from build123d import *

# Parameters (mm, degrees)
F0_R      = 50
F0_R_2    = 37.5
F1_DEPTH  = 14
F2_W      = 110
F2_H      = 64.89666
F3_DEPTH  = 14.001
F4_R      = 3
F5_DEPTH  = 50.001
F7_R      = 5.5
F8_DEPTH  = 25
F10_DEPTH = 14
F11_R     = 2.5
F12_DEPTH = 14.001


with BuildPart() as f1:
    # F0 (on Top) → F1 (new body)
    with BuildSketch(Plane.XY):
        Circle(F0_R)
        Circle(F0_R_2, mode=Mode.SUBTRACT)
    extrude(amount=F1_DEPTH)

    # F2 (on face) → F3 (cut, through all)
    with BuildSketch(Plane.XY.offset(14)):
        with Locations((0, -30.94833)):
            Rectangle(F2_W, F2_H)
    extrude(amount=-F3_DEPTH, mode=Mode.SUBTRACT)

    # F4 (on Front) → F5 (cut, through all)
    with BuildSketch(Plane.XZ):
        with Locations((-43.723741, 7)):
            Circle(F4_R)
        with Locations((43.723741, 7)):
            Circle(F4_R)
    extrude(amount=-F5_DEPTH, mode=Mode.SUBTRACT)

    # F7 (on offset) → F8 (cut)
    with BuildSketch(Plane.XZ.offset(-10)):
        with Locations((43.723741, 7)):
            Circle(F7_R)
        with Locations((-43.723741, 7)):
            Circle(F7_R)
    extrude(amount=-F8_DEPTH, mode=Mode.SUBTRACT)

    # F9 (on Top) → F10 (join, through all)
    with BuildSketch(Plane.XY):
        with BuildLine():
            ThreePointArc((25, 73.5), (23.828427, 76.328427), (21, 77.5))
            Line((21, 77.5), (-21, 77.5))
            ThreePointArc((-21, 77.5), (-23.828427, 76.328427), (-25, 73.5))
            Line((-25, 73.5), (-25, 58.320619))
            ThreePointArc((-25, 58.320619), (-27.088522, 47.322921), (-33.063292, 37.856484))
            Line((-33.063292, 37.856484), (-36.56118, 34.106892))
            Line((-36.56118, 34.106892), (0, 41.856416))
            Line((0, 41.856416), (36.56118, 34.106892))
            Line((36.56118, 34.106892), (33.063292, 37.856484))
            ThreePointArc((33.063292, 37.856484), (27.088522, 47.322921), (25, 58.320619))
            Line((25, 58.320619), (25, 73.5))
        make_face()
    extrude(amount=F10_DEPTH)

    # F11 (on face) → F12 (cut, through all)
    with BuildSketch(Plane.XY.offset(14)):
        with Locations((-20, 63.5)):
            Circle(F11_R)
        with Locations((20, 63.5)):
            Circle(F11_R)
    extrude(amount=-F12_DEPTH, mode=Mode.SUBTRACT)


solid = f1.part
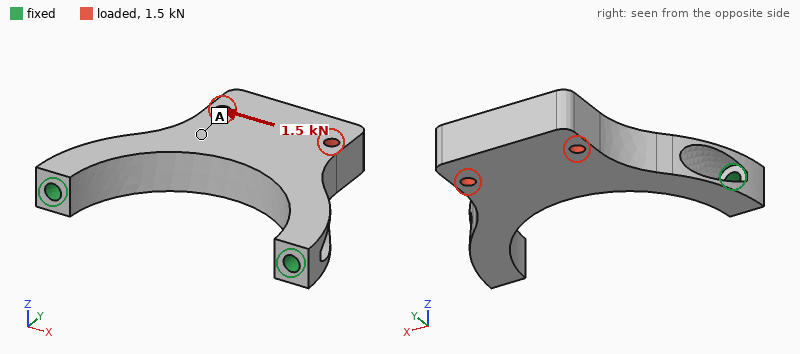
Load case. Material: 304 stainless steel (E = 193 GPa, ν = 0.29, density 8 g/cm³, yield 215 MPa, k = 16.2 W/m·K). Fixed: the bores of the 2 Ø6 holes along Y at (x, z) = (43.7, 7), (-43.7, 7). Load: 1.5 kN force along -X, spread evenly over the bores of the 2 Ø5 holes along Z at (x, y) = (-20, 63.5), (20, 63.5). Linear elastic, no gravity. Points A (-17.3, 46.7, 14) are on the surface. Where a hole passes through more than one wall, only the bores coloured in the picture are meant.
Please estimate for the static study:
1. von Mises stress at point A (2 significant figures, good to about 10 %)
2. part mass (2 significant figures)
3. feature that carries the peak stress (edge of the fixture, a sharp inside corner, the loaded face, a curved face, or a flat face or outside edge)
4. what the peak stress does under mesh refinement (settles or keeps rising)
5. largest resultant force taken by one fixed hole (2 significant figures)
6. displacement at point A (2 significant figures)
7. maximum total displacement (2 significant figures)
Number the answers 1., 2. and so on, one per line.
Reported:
1. 3.8 MPa
2. 330 g
3. edge of the fixture
4. keeps rising
5. 1.2 kN
6. 6.1 µm
7. 6.7 µm
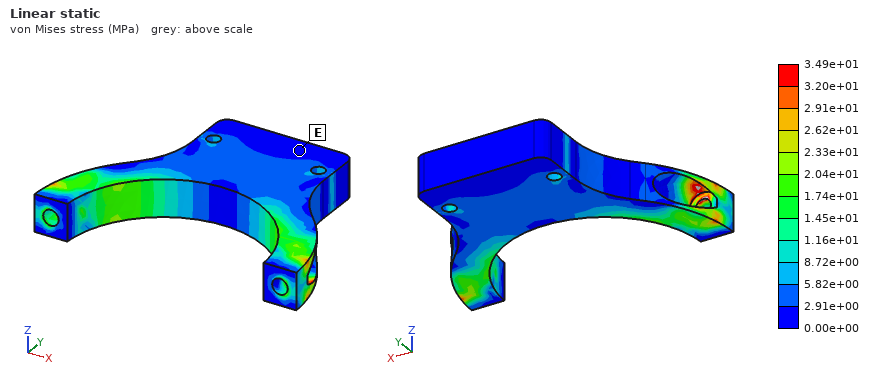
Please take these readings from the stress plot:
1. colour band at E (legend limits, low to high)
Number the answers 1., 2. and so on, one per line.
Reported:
1. 0.00e+00 to 2.91e+00 MPa
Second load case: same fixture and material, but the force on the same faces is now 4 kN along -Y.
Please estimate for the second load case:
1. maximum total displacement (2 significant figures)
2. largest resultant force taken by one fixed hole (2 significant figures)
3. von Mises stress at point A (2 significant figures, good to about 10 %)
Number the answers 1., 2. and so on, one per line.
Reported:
1. 7.1 µm
2. 2.2 kN
3. 6.9 MPa
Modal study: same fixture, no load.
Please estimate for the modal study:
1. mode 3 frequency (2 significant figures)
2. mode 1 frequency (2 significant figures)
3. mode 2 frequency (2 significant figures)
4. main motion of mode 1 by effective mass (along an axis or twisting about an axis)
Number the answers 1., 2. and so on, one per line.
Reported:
1. 4600 Hz
2. 1100 Hz
3. 4400 Hz
4. along Z
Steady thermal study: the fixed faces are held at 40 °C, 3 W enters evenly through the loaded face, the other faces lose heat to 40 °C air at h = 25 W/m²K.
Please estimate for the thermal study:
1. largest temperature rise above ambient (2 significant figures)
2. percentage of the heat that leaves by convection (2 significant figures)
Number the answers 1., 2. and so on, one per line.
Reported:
1. 14 K
2. 75 %
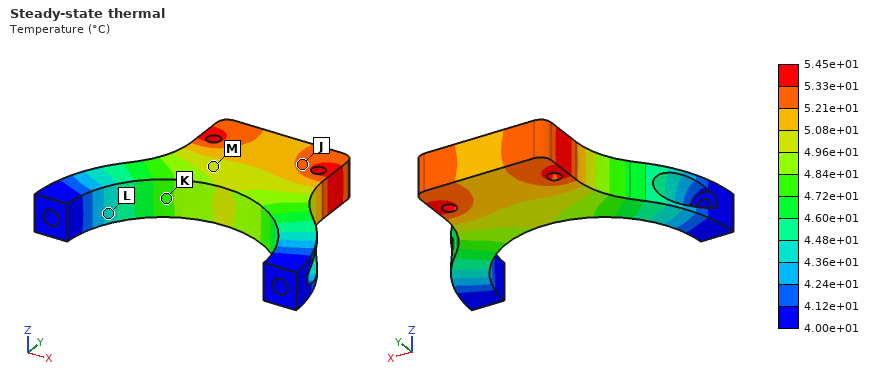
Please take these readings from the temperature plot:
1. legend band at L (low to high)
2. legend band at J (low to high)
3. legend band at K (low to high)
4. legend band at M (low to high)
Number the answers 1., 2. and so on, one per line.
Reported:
1. 4.36e+01 to 4.48e+01 °C
2. 5.21e+01 to 5.33e+01 °C
3. 4.72e+01 to 4.84e+01 °C
4. 4.96e+01 to 5.08e+01 °C
